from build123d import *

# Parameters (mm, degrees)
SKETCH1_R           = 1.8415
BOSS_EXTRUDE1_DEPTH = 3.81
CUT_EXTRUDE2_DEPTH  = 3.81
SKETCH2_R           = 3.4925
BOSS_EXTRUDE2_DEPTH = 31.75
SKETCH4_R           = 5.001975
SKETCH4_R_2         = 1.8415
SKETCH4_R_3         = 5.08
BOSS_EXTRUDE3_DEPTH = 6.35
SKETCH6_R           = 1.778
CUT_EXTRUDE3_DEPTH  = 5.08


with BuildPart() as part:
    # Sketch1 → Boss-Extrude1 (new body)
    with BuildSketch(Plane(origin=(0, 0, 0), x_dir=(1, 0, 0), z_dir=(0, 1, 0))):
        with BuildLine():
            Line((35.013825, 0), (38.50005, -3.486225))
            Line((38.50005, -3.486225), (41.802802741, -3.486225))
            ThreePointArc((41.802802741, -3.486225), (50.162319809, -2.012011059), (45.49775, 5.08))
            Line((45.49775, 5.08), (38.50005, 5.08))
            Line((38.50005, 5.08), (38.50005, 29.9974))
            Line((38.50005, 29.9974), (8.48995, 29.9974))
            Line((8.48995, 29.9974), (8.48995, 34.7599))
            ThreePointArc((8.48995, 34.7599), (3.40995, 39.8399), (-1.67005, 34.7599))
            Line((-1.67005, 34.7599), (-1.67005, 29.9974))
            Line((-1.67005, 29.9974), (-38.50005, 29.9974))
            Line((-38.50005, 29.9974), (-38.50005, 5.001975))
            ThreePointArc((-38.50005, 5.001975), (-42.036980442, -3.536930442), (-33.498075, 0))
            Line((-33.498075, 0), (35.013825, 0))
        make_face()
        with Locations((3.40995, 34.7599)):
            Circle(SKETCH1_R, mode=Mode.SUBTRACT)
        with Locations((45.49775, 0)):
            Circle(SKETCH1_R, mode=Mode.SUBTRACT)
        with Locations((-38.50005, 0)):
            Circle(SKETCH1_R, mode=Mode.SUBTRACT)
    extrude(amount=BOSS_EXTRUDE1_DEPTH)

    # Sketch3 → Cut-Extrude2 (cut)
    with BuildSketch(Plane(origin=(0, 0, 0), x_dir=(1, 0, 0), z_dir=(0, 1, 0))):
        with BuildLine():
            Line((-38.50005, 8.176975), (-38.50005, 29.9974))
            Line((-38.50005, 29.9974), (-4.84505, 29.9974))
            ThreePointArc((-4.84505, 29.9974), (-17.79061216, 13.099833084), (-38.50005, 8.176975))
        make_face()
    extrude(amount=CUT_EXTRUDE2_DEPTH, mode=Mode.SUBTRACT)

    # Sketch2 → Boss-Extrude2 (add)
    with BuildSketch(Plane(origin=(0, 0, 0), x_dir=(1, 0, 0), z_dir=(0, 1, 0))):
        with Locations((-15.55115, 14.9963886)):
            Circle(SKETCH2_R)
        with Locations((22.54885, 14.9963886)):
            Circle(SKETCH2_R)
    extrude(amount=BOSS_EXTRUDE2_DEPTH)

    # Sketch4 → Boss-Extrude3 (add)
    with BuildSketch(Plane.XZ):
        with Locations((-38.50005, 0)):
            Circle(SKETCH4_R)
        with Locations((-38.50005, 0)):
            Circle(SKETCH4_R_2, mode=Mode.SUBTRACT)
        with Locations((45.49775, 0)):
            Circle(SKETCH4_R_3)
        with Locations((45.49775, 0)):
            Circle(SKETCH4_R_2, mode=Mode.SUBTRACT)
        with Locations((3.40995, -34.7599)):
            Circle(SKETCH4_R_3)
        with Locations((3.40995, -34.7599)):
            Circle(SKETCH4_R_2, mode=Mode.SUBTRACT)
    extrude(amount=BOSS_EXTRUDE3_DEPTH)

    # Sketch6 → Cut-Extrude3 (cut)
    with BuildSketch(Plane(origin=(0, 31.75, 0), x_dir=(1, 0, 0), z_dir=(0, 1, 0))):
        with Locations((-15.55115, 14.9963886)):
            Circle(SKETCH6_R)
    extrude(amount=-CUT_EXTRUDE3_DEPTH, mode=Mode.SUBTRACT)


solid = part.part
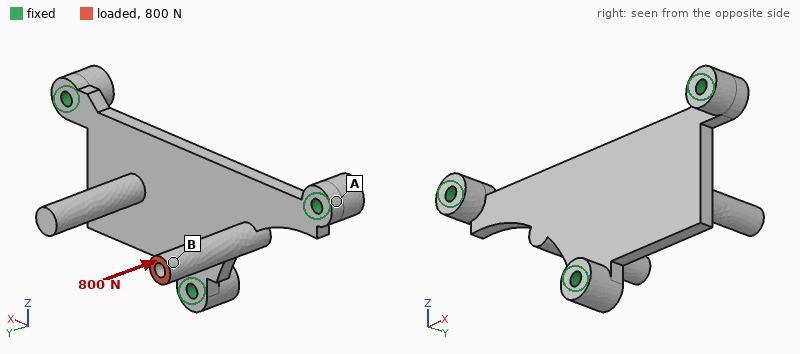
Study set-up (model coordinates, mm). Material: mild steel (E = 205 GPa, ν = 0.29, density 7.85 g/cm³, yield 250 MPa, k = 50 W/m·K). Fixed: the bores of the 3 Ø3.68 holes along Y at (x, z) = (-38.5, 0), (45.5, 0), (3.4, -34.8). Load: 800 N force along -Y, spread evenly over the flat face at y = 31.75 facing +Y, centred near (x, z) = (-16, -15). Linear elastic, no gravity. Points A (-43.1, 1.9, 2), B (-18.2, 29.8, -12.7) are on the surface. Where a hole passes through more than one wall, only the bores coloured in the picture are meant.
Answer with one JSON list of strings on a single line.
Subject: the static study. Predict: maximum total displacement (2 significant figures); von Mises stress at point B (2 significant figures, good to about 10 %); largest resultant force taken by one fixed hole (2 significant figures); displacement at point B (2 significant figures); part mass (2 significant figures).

["86 µm", "28 MPa", "440 N", "78 µm", "86 g"]
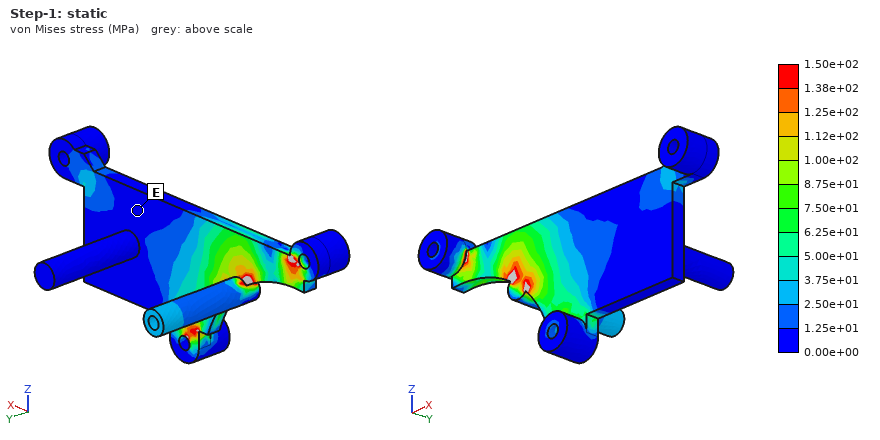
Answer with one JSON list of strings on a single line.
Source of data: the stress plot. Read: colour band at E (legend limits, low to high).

["0.00e+00 to 1.25e+01 MPa"]
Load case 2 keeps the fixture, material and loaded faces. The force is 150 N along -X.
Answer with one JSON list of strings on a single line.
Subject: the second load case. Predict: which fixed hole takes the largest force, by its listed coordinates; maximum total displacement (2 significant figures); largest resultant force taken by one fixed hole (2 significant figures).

["(-38.5, 0)", "0.13 mm", "130 N"]
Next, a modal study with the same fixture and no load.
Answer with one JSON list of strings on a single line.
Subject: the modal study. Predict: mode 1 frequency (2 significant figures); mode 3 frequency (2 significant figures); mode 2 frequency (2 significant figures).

["2600 Hz", "4200 Hz", "3300 Hz"]
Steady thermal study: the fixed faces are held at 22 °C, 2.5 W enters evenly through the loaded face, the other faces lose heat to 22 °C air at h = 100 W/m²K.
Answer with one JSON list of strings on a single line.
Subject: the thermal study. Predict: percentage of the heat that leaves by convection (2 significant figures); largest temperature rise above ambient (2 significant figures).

["75 %", "33 K"]
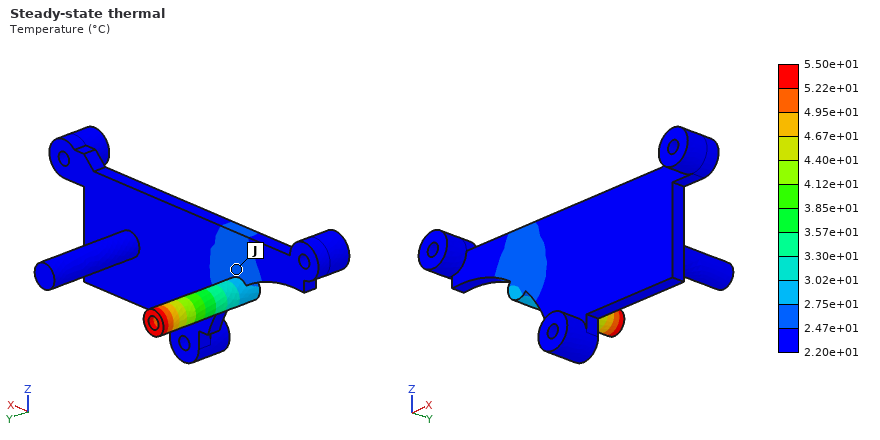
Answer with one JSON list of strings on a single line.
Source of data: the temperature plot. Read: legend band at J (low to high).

["2.47e+01 to 2.75e+01 °C"]
